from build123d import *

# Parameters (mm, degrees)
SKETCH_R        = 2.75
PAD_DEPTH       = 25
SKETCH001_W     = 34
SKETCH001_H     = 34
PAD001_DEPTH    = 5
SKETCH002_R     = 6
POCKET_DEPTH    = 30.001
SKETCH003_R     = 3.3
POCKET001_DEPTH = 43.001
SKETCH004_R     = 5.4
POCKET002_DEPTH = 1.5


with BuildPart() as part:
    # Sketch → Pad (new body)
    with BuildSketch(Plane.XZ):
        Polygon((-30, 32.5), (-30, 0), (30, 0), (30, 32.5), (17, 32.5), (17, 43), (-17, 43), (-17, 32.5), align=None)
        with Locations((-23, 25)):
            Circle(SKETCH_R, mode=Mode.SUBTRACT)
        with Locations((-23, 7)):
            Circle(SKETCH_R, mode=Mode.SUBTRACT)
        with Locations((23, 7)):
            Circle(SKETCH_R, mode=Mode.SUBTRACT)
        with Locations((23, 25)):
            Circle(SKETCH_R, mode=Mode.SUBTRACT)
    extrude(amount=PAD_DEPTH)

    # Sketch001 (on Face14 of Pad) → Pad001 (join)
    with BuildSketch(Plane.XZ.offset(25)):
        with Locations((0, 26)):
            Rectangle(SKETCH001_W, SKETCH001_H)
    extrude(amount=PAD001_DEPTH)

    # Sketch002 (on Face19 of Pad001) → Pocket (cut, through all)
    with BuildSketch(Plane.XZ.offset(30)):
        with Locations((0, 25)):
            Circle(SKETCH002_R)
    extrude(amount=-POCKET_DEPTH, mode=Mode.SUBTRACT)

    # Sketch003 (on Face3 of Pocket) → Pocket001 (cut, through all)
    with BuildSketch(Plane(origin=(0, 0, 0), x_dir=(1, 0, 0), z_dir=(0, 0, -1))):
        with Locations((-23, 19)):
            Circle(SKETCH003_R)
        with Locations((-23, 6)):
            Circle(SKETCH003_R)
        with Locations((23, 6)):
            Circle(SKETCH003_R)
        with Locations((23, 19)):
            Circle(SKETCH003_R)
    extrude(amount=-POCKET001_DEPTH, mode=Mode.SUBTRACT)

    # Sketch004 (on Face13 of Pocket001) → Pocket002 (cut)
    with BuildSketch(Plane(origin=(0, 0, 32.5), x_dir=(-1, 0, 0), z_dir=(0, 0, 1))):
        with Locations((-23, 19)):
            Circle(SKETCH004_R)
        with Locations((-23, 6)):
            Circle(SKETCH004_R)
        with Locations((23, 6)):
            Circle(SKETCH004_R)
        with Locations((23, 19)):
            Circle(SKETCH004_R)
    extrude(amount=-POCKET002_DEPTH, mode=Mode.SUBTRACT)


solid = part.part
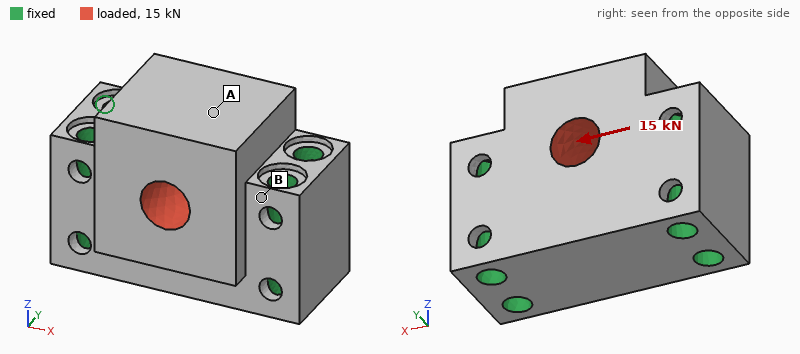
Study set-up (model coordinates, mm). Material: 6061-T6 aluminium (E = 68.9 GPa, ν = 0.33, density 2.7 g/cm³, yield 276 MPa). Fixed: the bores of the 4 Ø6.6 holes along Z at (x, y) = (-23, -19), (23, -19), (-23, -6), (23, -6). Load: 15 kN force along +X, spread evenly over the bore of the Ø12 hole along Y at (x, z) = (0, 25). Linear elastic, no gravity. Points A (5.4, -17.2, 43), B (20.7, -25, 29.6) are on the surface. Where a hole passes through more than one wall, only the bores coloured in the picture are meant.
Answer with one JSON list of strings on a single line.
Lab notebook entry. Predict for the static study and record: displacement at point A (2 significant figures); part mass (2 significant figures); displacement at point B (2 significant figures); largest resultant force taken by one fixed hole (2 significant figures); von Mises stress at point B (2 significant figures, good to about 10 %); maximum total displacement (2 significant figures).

["3.0 µm", "150 g", "1.3 µm", "4.2 kN", "15 MPa", "5.5 µm"]
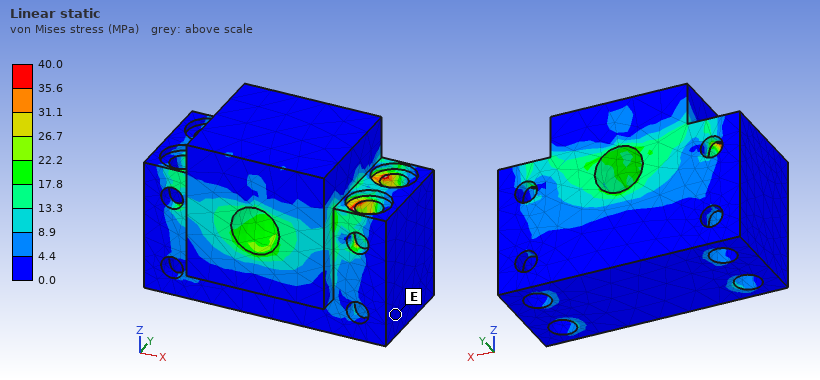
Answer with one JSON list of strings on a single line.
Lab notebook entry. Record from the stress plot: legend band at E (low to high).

["0.0 to 4.4 MPa"]
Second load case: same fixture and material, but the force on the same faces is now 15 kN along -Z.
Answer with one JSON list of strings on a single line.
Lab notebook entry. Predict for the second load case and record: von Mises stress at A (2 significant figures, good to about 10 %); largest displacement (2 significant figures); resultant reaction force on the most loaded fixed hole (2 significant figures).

["12 MPa", "9.7 µm", "4.5 kN"]
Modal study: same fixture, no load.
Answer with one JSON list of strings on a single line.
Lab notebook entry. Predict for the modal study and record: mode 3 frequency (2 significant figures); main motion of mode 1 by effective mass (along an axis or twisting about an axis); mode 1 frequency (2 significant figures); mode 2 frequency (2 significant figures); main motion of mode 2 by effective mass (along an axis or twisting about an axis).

["31 kHz", "along Y", "19 kHz", "29 kHz", "along Z"]
